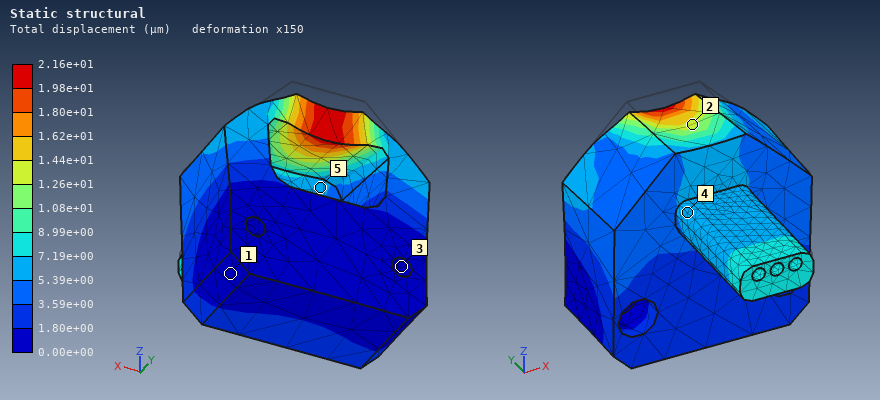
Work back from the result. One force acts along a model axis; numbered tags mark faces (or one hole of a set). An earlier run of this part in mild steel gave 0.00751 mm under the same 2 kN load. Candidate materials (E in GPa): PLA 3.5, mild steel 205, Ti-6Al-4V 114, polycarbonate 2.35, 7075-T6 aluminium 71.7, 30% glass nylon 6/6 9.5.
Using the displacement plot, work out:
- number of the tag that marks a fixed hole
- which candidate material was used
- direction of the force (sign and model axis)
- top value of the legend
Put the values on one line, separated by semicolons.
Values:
3; 7075-T6 aluminium; -Z; 2.16e+01 µm
